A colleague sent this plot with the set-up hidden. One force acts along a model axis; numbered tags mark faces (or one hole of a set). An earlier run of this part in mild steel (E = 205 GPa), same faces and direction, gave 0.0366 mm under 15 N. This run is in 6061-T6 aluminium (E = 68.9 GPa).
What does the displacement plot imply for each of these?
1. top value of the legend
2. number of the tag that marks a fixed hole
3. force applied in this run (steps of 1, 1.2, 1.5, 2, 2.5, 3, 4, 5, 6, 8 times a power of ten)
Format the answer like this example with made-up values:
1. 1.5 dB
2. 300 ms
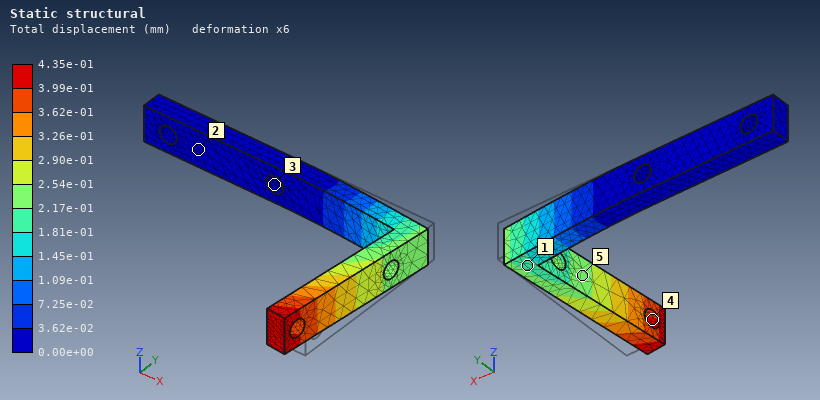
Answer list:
1. 4.35e-01 mm
2. 3
3. 60 N
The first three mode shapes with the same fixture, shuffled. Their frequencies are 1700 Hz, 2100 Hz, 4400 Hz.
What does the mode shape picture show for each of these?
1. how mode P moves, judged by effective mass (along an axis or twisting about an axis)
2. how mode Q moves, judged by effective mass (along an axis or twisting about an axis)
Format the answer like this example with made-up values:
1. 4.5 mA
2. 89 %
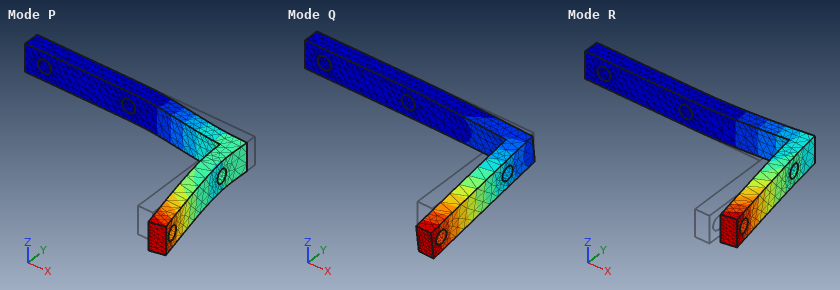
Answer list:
1. along Y
2. along Z
